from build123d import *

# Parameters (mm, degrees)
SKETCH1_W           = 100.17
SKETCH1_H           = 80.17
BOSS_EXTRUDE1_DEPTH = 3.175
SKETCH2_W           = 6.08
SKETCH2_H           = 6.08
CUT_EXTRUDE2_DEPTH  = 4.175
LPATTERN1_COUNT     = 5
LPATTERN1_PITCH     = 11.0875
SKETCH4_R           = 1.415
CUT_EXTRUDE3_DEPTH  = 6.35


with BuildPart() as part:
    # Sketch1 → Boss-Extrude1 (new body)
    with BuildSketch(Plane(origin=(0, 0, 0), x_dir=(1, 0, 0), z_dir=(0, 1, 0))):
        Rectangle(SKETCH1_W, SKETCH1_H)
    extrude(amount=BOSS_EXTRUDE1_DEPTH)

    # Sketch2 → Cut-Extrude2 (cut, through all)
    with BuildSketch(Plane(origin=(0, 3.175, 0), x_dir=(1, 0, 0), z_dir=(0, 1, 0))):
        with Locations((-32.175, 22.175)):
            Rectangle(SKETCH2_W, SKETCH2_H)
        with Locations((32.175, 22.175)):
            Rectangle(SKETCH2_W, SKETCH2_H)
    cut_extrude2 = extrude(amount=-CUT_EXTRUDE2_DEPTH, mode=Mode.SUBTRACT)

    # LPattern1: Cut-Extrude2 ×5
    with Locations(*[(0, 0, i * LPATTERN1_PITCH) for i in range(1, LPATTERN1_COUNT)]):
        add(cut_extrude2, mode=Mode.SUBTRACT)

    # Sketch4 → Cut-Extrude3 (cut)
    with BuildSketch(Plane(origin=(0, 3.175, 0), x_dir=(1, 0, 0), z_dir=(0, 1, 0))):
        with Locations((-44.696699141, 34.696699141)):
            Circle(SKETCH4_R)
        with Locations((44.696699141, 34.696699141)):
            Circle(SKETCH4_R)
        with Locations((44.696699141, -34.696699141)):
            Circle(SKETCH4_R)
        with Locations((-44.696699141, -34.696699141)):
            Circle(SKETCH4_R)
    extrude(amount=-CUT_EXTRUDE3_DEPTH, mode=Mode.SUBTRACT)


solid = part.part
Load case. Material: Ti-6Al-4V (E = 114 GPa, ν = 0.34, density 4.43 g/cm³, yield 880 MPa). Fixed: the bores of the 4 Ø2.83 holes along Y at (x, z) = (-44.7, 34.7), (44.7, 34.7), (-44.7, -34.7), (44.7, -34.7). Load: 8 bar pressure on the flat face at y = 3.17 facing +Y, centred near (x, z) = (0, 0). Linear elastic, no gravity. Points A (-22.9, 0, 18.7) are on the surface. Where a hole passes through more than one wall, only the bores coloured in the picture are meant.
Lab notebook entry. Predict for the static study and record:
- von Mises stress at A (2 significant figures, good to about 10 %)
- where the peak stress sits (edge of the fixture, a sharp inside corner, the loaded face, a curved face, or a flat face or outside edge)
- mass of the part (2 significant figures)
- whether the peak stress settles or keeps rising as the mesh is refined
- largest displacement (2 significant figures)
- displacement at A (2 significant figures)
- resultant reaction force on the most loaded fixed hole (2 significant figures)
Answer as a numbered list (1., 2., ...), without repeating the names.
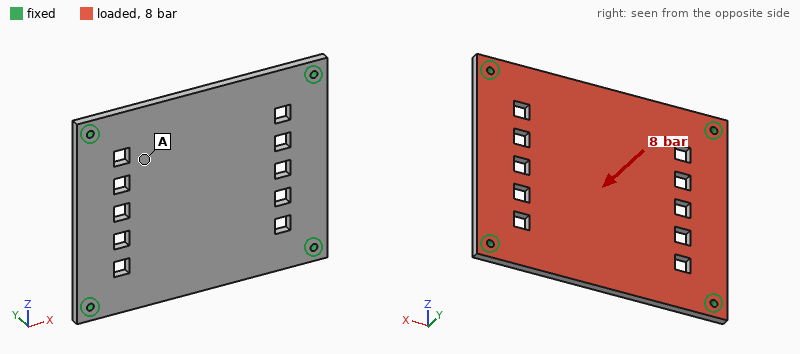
1. 110 MPa
2. edge of the fixture
3. 110 g
4. keeps rising
5. 0.87 mm
6. 0.56 mm
7. 1.5 kN
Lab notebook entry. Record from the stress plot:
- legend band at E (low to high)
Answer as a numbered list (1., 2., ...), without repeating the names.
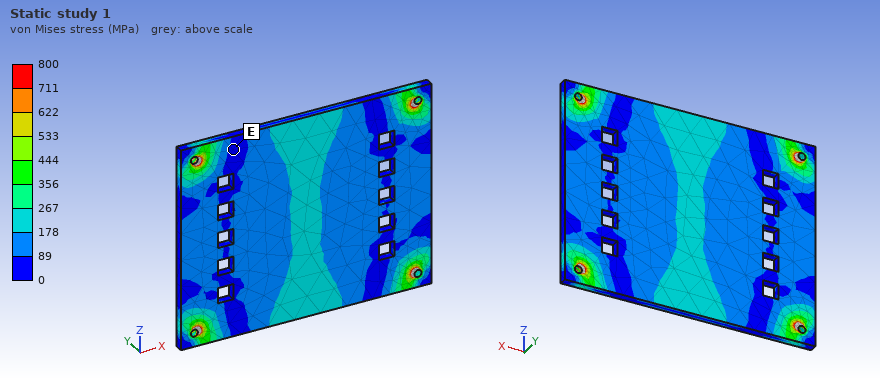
1. 0 to 89 MPa
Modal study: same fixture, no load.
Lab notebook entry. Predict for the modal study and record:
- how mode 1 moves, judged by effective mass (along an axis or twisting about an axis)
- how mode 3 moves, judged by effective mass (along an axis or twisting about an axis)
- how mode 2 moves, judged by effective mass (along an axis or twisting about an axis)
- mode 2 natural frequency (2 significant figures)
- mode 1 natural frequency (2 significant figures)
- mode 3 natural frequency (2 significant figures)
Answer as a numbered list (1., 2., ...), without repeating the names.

1. along Y
2. twisting about Z
3. twisting about X
4. 2400 Hz
5. 1500 Hz
6. 3200 Hz
